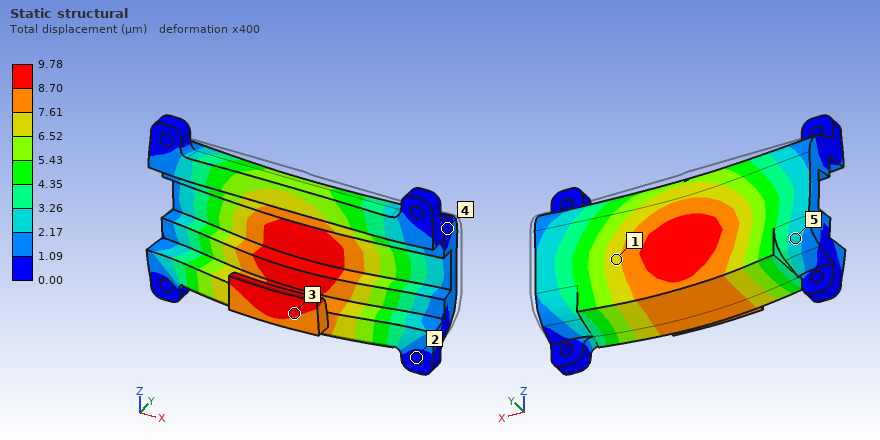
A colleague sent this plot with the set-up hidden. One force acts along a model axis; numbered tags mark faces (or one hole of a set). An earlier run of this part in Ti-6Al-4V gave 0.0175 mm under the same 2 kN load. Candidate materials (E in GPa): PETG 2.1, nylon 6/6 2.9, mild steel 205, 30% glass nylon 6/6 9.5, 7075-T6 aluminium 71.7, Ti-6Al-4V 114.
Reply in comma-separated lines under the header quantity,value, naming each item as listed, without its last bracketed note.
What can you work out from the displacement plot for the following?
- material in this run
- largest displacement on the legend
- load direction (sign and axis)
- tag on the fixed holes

quantity,value
material in this run,mild steel
largest displacement on the legend,9.78 µm
load direction,-Y
tag on the fixed holes,2
